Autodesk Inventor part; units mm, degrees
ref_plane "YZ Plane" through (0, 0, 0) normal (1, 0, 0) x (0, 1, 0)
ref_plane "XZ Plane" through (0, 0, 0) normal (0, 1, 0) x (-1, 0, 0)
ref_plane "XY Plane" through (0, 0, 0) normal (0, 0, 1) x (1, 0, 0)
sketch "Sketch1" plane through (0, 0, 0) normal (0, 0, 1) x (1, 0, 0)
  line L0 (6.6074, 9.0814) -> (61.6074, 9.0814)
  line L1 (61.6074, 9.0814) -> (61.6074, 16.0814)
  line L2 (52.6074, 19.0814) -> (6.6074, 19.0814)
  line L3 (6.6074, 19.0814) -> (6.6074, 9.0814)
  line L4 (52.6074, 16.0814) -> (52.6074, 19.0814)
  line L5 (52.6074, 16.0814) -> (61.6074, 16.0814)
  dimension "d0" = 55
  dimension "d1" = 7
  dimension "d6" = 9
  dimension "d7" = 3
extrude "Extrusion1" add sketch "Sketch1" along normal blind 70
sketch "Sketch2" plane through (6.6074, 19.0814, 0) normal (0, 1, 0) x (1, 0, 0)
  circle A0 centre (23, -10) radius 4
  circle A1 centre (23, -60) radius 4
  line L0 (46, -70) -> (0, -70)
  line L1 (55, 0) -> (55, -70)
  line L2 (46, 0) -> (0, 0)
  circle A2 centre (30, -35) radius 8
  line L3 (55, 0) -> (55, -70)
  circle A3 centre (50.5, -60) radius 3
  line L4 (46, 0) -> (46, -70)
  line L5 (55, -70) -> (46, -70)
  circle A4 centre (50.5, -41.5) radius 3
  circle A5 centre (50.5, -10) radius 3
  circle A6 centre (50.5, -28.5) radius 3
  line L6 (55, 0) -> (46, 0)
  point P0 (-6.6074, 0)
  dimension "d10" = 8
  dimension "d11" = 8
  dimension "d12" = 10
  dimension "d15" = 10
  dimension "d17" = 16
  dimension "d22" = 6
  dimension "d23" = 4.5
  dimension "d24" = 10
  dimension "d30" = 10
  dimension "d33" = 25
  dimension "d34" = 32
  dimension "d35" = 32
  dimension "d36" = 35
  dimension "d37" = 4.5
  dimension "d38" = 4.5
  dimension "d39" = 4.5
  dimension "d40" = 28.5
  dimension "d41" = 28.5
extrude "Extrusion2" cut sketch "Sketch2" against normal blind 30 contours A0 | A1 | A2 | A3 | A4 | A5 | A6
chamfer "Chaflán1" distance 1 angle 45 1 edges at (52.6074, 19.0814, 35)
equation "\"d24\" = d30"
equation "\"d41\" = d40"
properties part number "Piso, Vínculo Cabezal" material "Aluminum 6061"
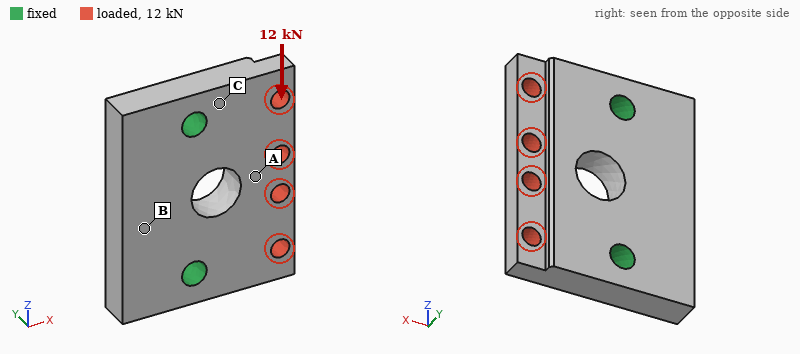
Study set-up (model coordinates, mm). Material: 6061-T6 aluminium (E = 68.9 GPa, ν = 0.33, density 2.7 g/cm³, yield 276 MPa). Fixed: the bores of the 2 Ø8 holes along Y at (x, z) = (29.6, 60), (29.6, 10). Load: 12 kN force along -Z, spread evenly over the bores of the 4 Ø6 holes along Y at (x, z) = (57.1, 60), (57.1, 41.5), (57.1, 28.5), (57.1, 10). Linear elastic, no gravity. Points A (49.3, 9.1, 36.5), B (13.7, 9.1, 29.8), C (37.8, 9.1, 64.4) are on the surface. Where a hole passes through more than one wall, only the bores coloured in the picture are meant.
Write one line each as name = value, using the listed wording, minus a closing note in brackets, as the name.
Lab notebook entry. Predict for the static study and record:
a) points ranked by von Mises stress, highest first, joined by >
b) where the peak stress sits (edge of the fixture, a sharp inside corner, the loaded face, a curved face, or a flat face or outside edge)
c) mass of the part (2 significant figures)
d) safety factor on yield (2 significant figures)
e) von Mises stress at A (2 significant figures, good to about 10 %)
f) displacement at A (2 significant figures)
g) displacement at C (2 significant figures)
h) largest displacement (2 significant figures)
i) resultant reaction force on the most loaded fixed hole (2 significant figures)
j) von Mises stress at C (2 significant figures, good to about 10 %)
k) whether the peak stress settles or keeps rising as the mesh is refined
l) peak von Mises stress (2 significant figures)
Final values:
points ranked by von Mises stress, highest first, joined by > = A > C > B
where the peak stress sits = the loaded face
mass of the part = 88 g
safety factor on yield = 1.9
von Mises stress at A = 68 MPa
displacement at A = 26 µm
displacement at C = 9.9 µm
largest displacement = 53 µm
resultant reaction force on the most loaded fixed hole = 8.1 kN
von Mises stress at C = 35 MPa
whether the peak stress settles or keeps rising as the mesh is refined = settles
peak von Mises stress = 140 MPa
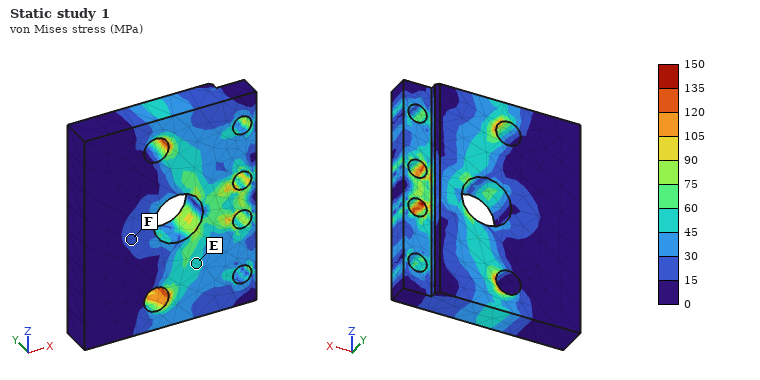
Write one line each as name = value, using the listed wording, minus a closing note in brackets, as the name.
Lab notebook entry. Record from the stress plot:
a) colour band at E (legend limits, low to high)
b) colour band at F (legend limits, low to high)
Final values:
colour band at E = 45 to 60 MPa
colour band at F = 15 to 30 MPa
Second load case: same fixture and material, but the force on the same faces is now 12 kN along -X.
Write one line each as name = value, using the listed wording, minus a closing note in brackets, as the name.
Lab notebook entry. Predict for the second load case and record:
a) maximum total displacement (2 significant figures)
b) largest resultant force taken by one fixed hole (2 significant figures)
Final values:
maximum total displacement = 41 µm
largest resultant force taken by one fixed hole = 6.1 kN
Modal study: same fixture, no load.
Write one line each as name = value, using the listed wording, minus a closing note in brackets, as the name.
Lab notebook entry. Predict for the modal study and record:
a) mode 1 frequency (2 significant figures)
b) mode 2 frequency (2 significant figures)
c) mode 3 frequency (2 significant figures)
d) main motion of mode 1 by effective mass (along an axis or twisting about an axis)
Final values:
mode 1 frequency = 7800 Hz
mode 2 frequency = 12 kHz
mode 3 frequency = 12 kHz
main motion of mode 1 by effective mass = along Y
